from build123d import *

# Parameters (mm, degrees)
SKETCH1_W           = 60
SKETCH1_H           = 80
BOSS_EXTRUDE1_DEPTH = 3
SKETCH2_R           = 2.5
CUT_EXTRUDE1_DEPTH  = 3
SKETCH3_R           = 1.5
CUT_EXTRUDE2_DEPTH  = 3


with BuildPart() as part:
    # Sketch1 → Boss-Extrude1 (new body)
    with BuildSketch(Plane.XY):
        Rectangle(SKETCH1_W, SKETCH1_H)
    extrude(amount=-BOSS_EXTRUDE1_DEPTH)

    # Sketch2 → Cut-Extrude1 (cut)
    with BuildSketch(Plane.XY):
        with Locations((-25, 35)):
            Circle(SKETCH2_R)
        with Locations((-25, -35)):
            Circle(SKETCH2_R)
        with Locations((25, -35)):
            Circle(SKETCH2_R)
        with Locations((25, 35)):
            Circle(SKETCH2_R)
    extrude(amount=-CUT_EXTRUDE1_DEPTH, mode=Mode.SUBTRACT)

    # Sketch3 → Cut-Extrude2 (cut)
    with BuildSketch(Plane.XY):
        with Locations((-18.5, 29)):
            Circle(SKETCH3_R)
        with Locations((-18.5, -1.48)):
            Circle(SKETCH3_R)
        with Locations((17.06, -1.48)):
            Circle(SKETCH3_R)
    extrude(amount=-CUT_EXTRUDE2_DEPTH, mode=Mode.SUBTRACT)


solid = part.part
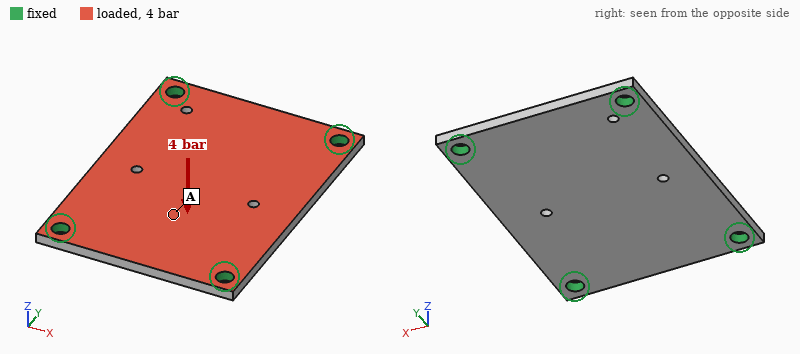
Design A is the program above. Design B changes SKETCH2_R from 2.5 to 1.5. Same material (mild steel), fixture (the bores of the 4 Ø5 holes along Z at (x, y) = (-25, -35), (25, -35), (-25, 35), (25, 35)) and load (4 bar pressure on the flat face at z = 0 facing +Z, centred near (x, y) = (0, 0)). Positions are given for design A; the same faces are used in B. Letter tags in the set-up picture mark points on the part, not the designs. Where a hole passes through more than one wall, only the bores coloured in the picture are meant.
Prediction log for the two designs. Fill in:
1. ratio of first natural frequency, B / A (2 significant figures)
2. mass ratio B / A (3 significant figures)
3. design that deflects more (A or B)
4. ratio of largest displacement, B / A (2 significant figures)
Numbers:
0.92
1.01
B
1.2
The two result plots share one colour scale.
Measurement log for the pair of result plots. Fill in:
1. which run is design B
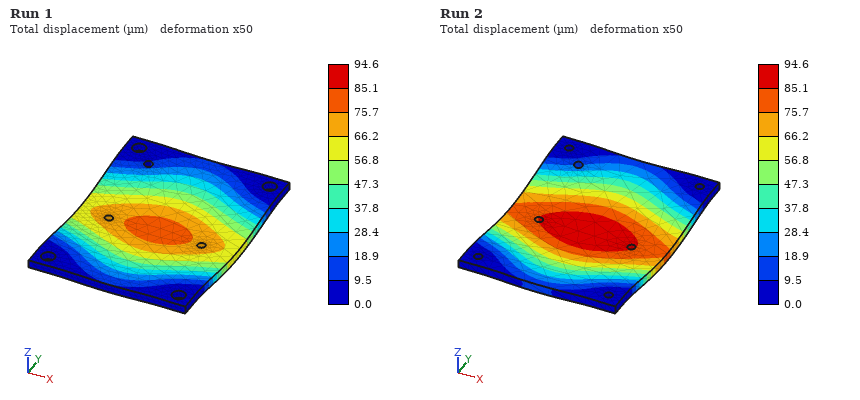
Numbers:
Run 2
